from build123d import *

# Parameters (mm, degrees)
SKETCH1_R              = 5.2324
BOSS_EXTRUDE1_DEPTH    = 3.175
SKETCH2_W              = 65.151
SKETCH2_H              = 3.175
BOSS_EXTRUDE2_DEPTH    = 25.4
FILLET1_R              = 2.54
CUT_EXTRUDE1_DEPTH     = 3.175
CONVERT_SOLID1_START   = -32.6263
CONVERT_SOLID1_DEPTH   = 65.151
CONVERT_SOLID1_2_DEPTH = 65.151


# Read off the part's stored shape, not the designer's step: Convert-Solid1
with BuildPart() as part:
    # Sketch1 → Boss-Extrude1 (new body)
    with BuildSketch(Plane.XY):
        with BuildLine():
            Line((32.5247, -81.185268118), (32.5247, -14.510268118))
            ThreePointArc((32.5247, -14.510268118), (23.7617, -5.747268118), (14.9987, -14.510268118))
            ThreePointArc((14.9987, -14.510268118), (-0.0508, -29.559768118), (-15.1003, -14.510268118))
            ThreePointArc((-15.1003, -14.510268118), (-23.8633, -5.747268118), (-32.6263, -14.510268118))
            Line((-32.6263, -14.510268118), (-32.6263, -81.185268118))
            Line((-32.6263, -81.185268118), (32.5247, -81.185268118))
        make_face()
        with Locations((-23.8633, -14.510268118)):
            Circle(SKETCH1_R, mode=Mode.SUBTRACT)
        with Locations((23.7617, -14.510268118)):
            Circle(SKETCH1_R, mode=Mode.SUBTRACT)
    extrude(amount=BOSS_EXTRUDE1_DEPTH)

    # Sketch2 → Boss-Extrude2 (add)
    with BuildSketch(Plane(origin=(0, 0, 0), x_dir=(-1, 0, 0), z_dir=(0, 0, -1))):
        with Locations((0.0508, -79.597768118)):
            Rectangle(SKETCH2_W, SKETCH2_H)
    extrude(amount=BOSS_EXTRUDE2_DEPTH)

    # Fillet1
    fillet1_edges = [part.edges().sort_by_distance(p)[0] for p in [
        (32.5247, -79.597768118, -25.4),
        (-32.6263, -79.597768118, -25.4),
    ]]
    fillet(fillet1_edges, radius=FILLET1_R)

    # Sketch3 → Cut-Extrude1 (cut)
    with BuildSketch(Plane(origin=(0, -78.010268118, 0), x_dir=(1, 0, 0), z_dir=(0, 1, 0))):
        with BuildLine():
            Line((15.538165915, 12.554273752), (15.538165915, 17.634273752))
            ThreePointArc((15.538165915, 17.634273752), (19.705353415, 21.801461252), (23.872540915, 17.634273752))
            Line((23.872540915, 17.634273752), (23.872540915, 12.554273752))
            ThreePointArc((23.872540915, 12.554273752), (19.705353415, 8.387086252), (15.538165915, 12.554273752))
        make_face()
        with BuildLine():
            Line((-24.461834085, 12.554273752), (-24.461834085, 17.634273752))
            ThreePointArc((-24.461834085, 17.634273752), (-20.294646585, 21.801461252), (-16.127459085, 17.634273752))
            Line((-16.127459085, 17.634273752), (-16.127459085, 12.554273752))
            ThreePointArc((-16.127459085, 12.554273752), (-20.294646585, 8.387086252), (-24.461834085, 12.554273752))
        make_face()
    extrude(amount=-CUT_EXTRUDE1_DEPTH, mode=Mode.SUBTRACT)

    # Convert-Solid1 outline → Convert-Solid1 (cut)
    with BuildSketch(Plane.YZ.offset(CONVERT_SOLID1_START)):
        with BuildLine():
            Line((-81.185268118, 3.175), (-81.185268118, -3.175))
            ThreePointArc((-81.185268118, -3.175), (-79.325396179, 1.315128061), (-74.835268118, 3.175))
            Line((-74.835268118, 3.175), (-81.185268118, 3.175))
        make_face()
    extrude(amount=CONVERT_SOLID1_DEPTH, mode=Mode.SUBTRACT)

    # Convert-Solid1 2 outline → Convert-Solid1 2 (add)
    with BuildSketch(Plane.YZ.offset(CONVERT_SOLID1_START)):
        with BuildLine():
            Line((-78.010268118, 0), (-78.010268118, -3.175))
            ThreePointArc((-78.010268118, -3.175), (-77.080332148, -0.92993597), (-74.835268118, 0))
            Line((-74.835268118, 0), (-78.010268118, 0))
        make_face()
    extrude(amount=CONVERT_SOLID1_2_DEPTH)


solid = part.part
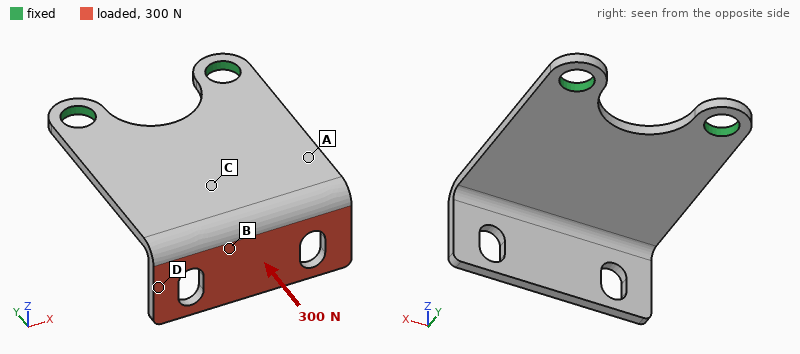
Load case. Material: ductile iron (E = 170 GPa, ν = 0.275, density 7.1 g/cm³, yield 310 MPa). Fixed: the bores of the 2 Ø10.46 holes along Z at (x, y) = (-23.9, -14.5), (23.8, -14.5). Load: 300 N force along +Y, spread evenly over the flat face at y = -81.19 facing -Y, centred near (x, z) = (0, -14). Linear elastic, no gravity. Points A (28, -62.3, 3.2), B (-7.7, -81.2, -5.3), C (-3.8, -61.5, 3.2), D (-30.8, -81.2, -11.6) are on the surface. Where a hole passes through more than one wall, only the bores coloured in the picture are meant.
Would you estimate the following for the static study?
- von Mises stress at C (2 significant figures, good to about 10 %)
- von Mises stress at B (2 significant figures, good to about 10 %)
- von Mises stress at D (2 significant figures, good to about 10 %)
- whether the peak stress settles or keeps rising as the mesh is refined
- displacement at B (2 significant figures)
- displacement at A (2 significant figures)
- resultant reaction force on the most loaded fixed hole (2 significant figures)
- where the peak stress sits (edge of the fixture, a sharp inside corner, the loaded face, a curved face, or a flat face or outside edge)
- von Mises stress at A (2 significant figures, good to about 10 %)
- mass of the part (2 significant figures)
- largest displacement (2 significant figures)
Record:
38 MPa
25 MPa
16 MPa
keeps rising
0.39 mm
0.20 mm
150 N
edge of the fixture
43 MPa
120 g
0.49 mm
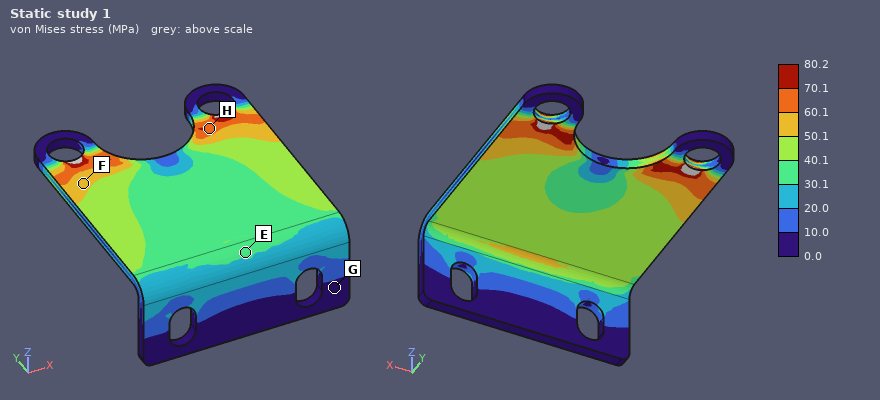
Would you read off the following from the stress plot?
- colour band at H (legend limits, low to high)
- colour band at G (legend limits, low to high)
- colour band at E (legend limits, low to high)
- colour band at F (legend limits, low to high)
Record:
60.1 to 70.1 MPa
0.0 to 10.0 MPa
30.1 to 40.1 MPa
50.1 to 60.1 MPa
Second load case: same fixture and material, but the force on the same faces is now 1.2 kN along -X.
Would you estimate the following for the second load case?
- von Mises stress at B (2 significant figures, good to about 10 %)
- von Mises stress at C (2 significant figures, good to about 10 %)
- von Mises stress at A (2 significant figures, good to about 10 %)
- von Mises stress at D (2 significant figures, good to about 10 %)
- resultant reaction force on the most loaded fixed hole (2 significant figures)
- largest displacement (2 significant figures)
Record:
56 MPa
100 MPa
120 MPa
36 MPa
1.6 kN
0.70 mm
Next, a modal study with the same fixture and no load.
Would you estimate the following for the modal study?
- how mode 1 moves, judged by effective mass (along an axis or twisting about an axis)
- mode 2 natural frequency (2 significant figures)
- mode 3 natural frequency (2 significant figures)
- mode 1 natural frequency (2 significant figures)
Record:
along Z
980 Hz
1800 Hz
360 Hz
